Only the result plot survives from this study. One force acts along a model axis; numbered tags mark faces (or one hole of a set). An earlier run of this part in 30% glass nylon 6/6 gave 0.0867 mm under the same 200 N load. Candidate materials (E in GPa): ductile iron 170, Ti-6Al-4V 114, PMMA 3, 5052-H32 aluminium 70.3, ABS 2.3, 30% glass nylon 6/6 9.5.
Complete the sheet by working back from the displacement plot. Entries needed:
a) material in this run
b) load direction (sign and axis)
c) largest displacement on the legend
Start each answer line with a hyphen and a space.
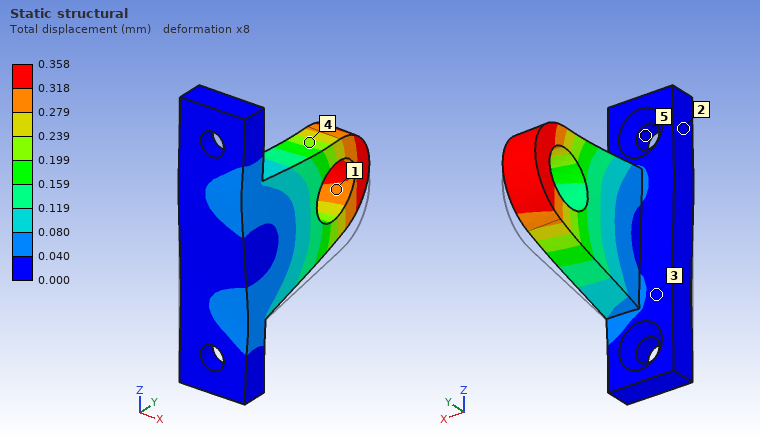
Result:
- ABS
- +Z
- 0.358 mm
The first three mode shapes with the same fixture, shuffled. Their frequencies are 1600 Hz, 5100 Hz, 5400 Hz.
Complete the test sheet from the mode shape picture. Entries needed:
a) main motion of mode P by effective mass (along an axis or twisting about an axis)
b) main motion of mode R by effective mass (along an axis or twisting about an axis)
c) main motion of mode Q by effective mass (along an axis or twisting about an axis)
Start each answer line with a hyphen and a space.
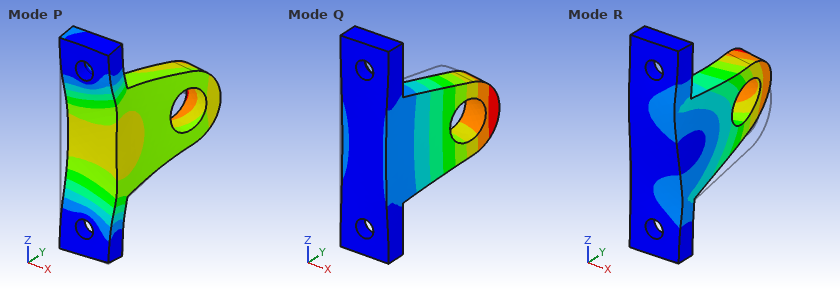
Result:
- along Y
- along Z
- along X
